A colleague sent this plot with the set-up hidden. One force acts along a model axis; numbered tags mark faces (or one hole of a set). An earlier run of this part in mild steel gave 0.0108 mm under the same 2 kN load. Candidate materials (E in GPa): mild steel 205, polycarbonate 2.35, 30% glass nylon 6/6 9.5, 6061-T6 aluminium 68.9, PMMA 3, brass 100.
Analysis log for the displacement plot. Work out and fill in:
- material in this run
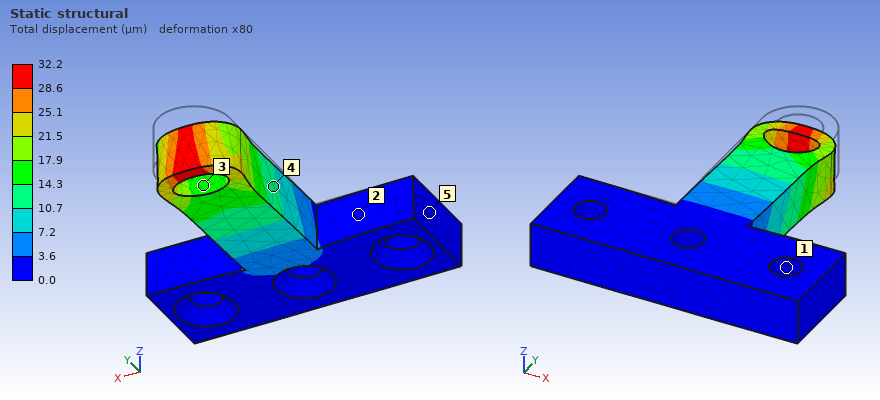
6061-T6 aluminium
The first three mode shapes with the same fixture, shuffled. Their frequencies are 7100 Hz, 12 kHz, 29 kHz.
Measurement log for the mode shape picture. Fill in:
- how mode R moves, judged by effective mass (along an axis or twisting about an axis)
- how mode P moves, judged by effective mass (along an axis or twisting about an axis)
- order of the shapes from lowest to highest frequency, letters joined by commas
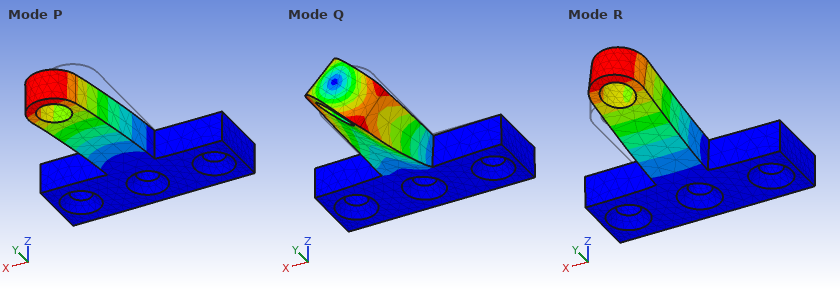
along Z
along X
R, P, Q
